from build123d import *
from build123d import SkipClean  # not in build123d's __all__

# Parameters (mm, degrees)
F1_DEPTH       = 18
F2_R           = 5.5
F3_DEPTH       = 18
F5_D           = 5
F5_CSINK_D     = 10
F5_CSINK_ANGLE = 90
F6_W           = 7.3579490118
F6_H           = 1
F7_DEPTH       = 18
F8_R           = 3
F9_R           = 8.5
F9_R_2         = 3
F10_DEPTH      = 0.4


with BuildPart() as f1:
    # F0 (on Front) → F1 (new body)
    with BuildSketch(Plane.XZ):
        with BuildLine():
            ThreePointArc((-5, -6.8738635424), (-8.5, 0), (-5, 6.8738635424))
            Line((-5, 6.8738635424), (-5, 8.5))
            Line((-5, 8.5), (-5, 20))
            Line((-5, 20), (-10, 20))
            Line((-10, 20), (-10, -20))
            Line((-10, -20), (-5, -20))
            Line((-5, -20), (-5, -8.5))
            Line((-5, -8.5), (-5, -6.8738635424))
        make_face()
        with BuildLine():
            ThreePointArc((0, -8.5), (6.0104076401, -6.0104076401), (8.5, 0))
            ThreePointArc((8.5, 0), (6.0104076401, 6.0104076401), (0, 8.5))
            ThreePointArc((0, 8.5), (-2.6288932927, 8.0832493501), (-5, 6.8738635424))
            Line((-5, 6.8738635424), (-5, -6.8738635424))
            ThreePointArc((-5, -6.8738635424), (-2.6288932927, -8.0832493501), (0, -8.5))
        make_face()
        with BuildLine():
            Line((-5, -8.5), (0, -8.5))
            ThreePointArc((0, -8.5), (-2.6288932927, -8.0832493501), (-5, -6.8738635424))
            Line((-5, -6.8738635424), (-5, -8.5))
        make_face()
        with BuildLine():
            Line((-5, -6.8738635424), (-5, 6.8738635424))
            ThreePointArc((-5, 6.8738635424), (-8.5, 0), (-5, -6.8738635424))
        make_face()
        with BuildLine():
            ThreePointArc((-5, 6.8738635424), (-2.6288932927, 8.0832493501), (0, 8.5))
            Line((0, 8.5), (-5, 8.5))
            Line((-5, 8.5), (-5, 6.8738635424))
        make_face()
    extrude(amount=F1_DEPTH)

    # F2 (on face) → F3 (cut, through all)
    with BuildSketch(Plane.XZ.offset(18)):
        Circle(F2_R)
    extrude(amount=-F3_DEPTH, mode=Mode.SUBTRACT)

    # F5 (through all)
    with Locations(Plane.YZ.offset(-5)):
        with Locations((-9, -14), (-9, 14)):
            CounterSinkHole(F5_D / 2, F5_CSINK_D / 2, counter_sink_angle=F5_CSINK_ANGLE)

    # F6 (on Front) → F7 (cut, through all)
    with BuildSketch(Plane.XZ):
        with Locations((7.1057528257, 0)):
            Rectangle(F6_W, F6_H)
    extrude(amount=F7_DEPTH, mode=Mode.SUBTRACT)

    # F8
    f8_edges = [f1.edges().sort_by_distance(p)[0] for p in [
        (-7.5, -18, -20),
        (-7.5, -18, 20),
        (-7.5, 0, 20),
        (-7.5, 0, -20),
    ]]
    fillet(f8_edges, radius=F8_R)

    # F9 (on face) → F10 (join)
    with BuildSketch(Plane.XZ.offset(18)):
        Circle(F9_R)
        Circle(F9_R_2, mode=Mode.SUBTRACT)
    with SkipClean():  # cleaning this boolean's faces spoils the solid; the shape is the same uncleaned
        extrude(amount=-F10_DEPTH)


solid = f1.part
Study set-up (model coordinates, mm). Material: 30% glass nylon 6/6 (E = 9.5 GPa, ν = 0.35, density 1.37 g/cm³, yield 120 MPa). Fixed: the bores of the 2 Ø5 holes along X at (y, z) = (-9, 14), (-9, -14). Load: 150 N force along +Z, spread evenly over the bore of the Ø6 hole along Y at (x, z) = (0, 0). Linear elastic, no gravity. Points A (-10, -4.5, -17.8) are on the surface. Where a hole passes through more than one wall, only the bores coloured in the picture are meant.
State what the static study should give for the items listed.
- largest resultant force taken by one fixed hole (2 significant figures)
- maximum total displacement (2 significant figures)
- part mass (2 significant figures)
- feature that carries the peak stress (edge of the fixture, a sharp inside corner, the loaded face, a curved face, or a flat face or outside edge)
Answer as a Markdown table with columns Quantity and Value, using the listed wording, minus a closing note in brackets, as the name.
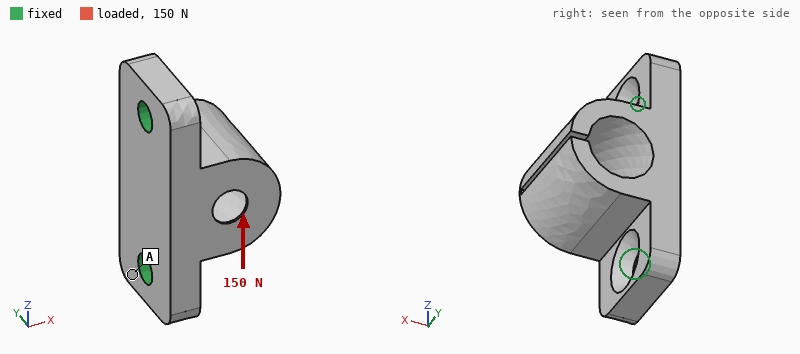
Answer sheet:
| Quantity | Value |
|---|---|
| largest resultant force taken by one fixed hole | 100 N |
| maximum total displacement | 34 µm |
| part mass | 6.9 g |
| feature that carries the peak stress | a curved face |
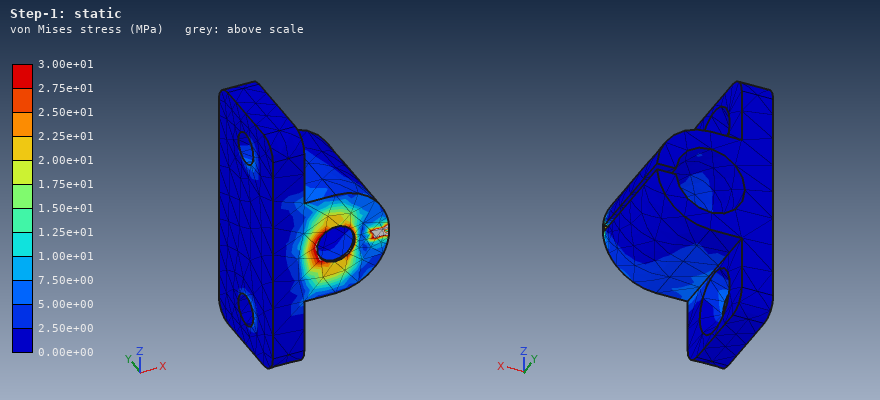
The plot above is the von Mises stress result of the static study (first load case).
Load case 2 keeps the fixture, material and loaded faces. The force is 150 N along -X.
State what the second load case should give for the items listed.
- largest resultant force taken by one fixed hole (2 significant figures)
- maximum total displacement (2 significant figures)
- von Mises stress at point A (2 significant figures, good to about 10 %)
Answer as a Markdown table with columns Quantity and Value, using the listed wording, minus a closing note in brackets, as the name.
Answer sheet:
| Quantity | Value |
|---|---|
| largest resultant force taken by one fixed hole | 92 N |
| maximum total displacement | 62 µm |
| von Mises stress at point A | 3.0 MPa |
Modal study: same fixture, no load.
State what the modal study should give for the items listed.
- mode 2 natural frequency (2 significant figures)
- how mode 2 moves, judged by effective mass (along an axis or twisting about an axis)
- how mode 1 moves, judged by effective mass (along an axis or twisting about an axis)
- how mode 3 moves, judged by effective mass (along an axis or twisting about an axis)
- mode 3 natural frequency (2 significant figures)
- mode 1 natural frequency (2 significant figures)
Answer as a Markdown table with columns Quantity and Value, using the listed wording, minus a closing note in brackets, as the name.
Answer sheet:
| Quantity | Value |
|---|---|
| mode 2 natural frequency | 6900 Hz |
| how mode 2 moves, judged by effective mass | along X |
| how mode 1 moves, judged by effective mass | along Y |
| how mode 3 moves, judged by effective mass | along Z |
| mode 3 natural frequency | 7900 Hz |
| mode 1 natural frequency | 5100 Hz |
